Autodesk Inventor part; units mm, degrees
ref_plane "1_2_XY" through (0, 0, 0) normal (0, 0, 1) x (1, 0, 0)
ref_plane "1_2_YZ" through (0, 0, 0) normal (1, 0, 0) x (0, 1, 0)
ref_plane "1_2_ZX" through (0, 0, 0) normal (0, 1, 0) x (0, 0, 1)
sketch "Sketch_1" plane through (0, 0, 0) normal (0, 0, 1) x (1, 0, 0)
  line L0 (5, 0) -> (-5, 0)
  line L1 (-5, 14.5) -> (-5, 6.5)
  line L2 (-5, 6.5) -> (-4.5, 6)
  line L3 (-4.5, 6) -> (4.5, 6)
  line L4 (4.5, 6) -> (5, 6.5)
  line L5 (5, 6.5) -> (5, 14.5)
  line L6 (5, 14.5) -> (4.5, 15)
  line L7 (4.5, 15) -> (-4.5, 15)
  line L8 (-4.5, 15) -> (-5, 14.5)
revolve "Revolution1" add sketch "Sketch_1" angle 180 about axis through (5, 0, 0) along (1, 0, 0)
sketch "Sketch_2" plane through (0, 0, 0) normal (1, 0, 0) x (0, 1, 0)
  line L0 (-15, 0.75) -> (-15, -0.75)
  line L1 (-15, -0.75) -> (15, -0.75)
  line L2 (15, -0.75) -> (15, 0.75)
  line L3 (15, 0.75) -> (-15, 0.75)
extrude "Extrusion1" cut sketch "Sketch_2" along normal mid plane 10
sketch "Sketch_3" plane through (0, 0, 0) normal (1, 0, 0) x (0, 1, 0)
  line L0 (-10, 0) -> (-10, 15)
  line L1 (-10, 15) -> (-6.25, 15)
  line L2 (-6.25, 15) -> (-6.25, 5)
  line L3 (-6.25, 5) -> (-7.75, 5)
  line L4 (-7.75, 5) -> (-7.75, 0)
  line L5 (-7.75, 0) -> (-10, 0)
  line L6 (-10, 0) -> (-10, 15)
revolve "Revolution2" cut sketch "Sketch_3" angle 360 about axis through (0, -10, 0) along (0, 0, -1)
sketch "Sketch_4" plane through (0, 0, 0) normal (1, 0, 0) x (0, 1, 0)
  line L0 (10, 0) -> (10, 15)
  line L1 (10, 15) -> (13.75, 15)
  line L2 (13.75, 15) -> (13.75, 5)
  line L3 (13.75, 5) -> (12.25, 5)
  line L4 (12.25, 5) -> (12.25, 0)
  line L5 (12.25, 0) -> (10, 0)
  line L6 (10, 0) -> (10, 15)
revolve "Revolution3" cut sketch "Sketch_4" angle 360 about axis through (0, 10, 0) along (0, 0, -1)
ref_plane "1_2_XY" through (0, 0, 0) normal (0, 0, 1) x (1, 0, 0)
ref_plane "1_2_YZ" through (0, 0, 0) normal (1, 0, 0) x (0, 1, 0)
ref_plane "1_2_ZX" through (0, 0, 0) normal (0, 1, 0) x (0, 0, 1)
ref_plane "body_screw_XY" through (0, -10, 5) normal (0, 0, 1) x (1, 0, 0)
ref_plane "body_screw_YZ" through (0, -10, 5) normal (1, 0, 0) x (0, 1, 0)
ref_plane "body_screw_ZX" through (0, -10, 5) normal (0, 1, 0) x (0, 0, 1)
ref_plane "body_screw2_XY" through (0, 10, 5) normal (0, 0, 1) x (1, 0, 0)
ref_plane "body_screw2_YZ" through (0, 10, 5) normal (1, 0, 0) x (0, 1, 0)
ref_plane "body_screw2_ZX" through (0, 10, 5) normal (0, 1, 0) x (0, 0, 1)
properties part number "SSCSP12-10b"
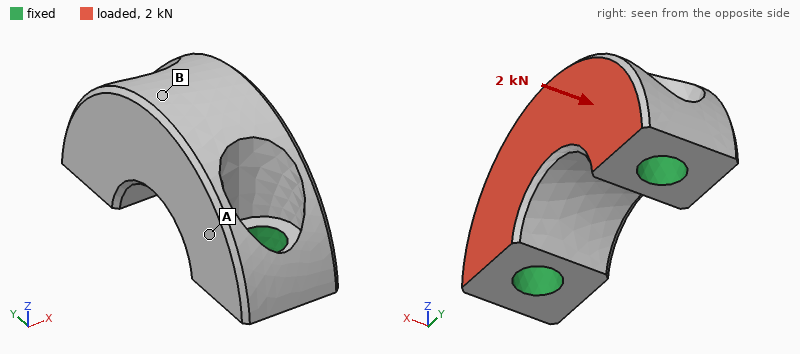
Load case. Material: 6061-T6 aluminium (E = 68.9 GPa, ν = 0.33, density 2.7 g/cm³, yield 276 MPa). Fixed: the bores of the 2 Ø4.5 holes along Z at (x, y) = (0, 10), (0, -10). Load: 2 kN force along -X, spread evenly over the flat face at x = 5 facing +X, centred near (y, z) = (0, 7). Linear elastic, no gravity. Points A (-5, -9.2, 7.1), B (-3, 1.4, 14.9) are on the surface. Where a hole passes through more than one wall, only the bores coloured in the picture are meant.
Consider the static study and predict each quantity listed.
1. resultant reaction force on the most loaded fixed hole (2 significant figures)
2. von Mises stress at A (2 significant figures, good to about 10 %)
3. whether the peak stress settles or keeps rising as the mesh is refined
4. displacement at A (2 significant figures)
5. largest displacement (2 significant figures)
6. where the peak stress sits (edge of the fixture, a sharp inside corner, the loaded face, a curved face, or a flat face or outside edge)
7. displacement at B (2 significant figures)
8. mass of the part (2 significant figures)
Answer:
1.0 kN
32 MPa
keeps rising
8.7 µm
25 µm
edge of the fixture
24 µm
5.8 g
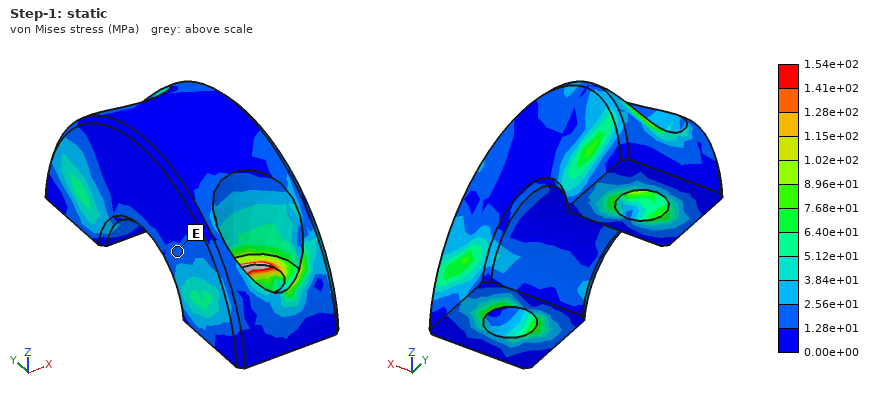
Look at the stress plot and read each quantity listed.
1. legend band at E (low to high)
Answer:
1.28e+01 to 2.56e+01 MPa
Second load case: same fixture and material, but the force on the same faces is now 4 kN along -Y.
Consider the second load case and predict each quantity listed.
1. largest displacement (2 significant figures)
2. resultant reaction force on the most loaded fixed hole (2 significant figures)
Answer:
21 µm
2.2 kN
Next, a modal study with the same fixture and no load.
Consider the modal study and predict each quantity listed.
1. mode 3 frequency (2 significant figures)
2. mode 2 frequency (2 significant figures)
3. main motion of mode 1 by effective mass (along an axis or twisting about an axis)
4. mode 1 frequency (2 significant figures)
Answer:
50 kHz
49 kHz
along X
22 kHz
